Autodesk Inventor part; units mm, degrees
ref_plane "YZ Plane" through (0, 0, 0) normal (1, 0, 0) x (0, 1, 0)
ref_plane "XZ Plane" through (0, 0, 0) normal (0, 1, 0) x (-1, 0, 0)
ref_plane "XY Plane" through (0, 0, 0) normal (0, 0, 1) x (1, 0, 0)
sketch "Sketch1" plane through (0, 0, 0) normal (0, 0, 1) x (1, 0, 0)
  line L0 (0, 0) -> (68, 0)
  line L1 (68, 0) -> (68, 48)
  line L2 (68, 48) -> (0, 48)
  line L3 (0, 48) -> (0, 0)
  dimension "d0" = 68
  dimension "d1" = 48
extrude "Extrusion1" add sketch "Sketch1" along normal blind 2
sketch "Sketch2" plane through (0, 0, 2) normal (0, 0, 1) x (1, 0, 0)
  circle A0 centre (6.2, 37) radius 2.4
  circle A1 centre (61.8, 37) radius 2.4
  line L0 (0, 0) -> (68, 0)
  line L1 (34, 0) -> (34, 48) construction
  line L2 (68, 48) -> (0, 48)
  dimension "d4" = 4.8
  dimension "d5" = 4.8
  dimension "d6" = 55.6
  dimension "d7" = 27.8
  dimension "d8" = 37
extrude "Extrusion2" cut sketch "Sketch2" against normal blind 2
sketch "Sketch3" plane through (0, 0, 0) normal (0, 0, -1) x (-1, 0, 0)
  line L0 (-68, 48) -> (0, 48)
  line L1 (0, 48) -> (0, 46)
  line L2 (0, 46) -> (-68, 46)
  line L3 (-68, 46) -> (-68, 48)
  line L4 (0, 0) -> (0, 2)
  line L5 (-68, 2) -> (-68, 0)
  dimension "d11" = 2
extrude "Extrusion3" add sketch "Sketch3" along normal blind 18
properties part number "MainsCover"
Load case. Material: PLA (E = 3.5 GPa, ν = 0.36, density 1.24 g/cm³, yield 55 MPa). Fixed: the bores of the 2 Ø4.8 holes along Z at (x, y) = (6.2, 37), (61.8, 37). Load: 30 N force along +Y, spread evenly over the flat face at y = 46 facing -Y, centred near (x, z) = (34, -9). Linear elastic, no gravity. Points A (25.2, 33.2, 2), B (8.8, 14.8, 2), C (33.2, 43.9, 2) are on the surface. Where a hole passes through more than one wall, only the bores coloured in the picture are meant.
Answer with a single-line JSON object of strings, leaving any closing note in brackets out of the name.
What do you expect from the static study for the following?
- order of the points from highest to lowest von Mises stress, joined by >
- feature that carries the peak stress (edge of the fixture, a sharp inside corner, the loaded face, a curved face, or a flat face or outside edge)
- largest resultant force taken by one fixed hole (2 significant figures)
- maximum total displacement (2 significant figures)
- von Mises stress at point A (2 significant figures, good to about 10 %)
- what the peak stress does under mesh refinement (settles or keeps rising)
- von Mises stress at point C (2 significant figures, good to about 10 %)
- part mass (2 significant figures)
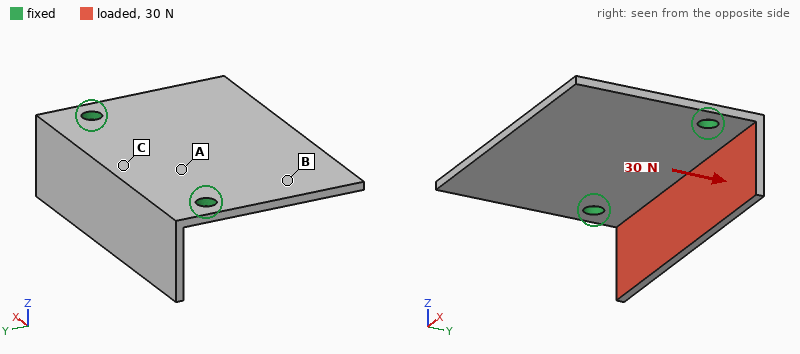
{"order of the points from highest to lowest von Mises stress, joined by >": "C > A > B", "feature that carries the peak stress": "edge of the fixture", "largest resultant force taken by one fixed hole": "15 N", "maximum total displacement": "0.53 mm", "von Mises stress at point A": "1.8 MPa", "what the peak stress does under mesh refinement": "keeps rising", "von Mises stress at point C": "4.4 MPa", "part mass": "11 g"}
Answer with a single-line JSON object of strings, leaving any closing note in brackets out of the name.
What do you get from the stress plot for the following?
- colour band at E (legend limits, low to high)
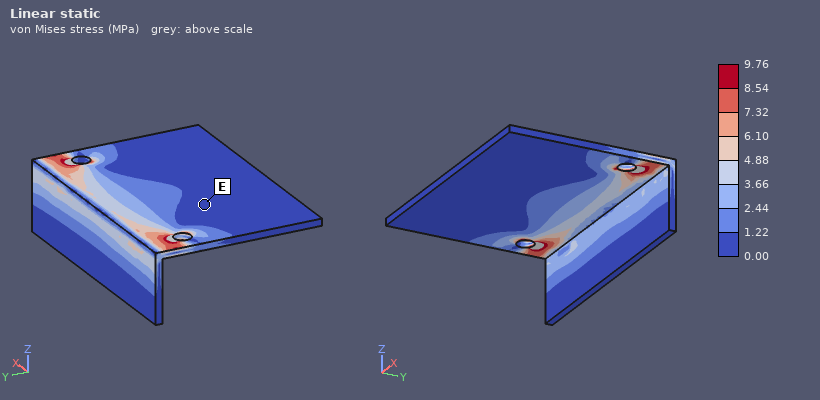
{"colour band at E": "0.00 to 1.22 MPa"}
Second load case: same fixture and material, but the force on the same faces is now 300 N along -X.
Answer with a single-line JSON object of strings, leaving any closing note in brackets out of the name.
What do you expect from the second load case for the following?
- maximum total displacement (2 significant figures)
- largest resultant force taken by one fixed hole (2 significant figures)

{"maximum total displacement": "0.82 mm", "largest resultant force taken by one fixed hole": "170 N"}
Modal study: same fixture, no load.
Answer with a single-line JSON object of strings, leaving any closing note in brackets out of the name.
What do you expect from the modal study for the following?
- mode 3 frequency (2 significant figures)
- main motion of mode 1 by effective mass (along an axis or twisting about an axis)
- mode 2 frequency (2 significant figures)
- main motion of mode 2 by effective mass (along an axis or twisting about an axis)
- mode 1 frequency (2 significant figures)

{"mode 3 frequency": "830 Hz", "main motion of mode 1 by effective mass": "along Z", "mode 2 frequency": "670 Hz", "main motion of mode 2 by effective mass": "twisting about Y", "mode 1 frequency": "350 Hz"}
